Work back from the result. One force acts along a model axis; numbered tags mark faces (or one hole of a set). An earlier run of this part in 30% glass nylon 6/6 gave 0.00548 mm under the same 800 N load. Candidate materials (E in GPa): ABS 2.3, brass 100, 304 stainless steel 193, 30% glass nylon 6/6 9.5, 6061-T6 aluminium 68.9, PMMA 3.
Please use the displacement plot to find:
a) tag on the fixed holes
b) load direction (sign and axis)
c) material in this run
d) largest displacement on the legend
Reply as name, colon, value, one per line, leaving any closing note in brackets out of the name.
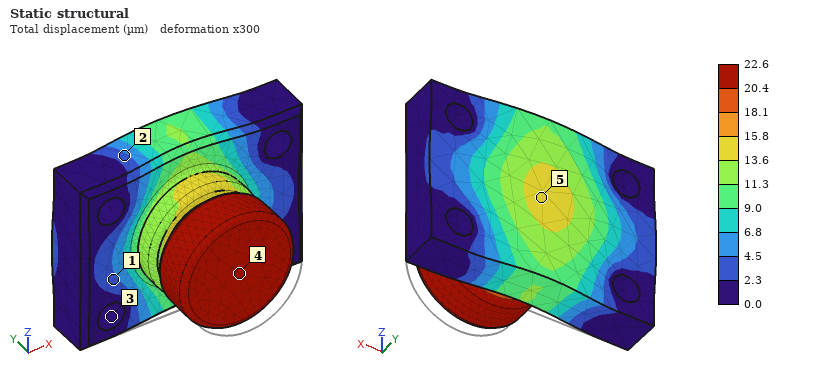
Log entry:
tag on the fixed holes: 3
load direction: +Y
material in this run: ABS
largest displacement on the legend: 22.6 µm
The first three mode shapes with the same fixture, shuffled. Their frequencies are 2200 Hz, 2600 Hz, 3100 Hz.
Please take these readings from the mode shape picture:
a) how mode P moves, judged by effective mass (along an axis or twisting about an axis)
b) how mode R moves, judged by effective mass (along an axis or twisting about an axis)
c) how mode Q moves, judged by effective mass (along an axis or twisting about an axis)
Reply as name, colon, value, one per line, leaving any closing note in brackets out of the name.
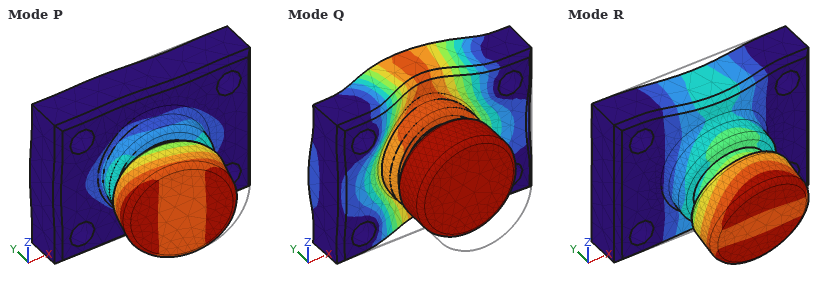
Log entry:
how mode P moves, judged by effective mass: along X
how mode R moves, judged by effective mass: along Z
how mode Q moves, judged by effective mass: along Y
